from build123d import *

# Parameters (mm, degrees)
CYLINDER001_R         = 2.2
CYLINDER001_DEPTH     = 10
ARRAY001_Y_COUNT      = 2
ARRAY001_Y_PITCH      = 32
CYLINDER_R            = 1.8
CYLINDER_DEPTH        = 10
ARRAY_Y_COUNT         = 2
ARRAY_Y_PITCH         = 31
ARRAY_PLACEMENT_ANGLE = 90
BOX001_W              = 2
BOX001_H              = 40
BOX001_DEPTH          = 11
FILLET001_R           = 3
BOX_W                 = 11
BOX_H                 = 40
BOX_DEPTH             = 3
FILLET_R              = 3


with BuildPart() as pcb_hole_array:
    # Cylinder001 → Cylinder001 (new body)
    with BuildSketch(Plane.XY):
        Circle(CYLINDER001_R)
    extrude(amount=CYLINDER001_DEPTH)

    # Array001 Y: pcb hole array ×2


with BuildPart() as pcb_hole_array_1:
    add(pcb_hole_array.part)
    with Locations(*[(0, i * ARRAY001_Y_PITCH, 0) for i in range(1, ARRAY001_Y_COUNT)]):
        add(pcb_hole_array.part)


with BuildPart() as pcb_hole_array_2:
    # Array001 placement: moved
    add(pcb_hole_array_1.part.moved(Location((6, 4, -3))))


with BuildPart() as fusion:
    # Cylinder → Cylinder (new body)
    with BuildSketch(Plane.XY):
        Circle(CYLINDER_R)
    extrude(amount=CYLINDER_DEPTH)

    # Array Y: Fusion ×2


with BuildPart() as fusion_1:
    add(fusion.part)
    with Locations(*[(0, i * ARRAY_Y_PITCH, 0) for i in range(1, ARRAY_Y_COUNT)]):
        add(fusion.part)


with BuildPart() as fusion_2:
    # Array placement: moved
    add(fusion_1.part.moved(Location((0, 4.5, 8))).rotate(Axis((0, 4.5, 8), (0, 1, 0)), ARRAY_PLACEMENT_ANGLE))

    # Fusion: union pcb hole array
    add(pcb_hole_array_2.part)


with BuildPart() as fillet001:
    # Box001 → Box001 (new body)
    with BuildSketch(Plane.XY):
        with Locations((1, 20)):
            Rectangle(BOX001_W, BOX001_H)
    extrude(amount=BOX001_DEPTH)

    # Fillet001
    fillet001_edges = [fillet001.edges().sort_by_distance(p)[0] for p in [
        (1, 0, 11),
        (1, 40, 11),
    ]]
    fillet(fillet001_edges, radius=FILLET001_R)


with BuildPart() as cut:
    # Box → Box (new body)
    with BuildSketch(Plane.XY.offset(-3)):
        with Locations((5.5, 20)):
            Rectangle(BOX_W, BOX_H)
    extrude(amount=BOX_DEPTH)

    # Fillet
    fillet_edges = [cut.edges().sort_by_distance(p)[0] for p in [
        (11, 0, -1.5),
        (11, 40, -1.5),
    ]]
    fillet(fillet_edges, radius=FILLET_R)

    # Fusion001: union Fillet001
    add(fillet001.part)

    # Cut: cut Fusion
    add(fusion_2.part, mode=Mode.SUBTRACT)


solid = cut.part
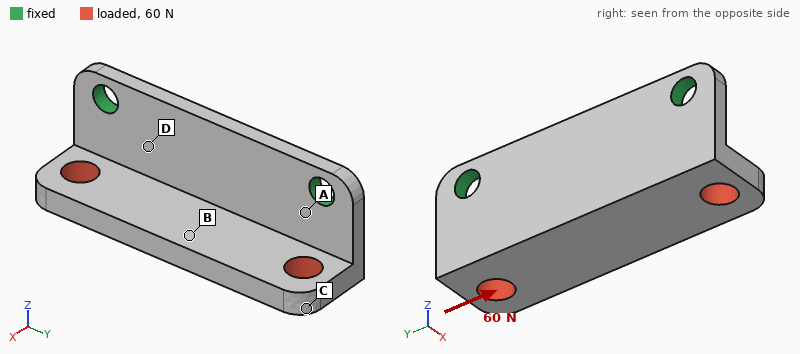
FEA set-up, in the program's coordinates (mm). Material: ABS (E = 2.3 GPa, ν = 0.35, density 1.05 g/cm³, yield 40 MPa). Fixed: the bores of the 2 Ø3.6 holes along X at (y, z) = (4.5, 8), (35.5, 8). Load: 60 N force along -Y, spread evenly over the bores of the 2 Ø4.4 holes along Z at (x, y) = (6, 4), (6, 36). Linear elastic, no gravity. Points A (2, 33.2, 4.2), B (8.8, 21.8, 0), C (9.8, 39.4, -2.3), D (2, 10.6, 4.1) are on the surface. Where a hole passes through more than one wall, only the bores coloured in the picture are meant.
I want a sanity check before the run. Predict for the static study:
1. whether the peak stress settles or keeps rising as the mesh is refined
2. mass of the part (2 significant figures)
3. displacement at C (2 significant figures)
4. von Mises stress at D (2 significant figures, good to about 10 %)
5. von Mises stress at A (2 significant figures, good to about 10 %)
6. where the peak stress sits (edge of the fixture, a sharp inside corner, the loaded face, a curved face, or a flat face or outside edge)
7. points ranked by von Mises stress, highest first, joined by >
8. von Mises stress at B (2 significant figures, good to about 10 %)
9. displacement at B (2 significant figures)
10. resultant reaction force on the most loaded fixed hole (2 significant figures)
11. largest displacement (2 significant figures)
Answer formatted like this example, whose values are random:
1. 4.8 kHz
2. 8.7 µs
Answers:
1. keeps rising
2. 2.2 g
3. 95 µm
4. 3.0 MPa
5. 3.6 MPa
6. edge of the fixture
7. A > D > B > C
8. 1.5 MPa
9. 44 µm
10. 35 N
11. 97 µm
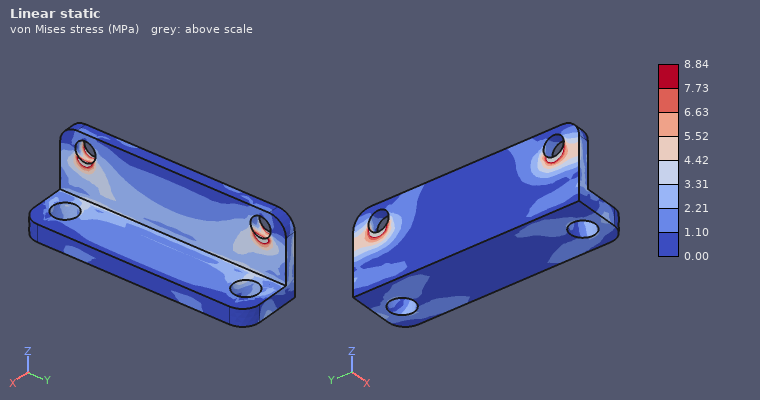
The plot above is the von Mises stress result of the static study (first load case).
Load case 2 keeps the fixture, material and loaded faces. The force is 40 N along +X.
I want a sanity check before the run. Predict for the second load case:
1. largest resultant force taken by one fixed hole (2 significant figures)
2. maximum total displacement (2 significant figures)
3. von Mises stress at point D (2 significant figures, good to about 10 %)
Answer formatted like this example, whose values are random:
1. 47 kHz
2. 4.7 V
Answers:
1. 20 N
2. 0.42 mm
3. 6.0 MPa
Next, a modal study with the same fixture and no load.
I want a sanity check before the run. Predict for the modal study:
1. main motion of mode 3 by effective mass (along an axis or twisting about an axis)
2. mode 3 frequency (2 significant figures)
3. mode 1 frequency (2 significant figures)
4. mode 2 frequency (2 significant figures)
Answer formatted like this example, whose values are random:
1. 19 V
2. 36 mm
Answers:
1. along X
2. 3800 Hz
3. 1400 Hz
4. 2800 Hz
